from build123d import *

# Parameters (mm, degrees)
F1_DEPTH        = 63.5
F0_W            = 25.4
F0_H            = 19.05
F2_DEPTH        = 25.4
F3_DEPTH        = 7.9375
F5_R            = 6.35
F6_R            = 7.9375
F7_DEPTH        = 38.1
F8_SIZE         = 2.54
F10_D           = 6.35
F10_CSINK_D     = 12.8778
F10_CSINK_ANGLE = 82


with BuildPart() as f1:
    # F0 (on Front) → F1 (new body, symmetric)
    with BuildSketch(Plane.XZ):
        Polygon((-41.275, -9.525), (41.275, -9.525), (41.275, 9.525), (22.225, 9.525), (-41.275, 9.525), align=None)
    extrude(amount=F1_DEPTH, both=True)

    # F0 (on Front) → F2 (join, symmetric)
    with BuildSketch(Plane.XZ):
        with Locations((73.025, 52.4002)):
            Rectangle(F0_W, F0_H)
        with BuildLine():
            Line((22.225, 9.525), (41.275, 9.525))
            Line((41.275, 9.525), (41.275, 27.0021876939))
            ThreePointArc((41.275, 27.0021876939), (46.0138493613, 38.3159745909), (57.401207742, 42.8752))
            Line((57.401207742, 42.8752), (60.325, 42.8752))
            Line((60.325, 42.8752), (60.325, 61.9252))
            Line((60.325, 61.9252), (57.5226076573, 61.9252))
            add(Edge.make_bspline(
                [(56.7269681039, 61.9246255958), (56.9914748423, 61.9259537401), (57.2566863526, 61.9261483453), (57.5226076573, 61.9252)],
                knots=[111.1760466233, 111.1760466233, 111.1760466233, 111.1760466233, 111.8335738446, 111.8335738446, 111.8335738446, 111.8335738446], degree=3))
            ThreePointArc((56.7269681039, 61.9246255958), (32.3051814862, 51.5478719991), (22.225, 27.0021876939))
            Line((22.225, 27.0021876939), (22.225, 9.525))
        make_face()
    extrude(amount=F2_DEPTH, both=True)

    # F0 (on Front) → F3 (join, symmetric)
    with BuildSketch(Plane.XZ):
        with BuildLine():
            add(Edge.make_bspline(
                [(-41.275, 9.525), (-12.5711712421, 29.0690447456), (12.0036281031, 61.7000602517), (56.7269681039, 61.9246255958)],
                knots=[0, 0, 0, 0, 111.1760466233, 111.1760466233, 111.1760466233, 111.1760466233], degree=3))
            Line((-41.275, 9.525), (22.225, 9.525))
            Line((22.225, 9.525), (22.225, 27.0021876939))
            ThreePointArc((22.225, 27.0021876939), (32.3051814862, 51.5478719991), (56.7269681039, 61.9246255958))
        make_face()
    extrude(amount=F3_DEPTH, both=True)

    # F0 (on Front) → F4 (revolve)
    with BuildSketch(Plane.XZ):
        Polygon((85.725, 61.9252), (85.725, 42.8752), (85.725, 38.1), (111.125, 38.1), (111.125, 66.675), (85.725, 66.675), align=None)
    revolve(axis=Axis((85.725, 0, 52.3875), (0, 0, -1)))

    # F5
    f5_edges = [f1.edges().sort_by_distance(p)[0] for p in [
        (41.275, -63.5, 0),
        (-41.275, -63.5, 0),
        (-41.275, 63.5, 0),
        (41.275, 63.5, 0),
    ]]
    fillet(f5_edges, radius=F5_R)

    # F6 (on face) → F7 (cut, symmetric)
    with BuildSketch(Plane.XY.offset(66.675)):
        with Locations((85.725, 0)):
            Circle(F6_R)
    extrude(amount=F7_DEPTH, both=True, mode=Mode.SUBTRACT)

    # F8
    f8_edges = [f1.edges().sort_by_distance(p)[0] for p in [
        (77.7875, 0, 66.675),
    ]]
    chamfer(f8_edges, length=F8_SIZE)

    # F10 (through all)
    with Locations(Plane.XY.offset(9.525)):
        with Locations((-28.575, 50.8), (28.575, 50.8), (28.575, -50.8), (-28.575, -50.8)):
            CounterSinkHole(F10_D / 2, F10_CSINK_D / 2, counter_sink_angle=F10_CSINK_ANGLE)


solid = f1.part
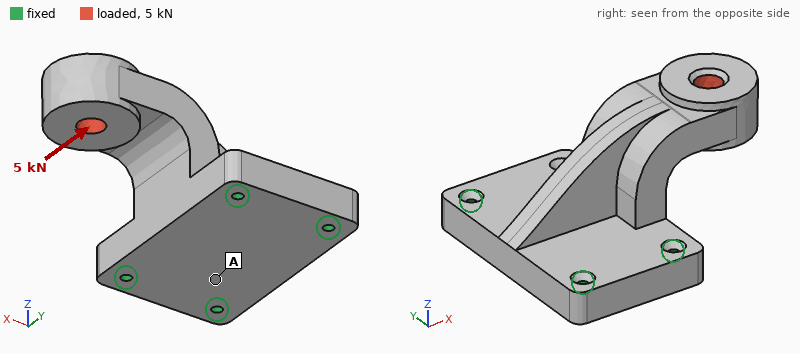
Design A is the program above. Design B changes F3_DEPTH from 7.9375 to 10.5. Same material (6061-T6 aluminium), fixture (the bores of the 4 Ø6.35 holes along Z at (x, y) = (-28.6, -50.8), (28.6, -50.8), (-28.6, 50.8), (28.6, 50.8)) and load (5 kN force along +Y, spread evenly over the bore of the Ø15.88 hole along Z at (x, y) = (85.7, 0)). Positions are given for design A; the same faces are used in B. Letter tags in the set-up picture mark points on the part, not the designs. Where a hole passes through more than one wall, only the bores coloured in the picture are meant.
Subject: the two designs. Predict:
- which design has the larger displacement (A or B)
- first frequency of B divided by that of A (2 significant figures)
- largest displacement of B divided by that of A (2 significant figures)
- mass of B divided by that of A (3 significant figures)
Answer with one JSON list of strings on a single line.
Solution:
["A", "1.0", "0.88", "1.03"]
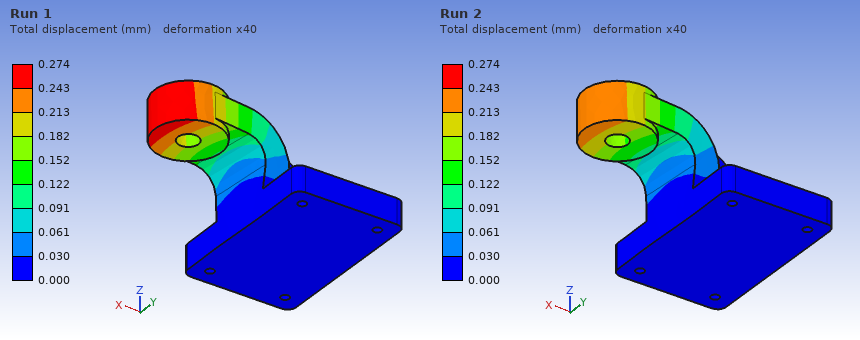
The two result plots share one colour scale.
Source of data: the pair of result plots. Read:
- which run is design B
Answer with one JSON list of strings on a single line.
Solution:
["Run 2"]
